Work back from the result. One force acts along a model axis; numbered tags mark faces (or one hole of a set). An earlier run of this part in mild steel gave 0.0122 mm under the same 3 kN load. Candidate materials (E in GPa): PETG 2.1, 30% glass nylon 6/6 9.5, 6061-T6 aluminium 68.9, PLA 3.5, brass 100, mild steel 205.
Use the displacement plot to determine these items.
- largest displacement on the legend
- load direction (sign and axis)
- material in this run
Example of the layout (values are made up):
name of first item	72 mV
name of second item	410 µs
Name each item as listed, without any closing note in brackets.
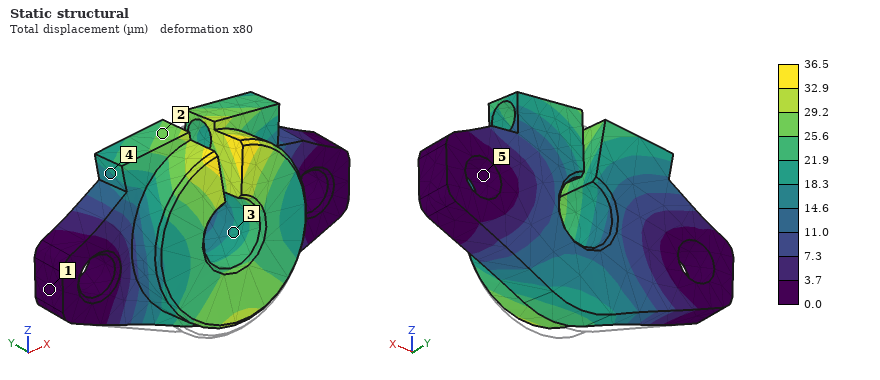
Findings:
largest displacement on the legend	36.5 µm
load direction	+Z
material in this run	6061-T6 aluminium
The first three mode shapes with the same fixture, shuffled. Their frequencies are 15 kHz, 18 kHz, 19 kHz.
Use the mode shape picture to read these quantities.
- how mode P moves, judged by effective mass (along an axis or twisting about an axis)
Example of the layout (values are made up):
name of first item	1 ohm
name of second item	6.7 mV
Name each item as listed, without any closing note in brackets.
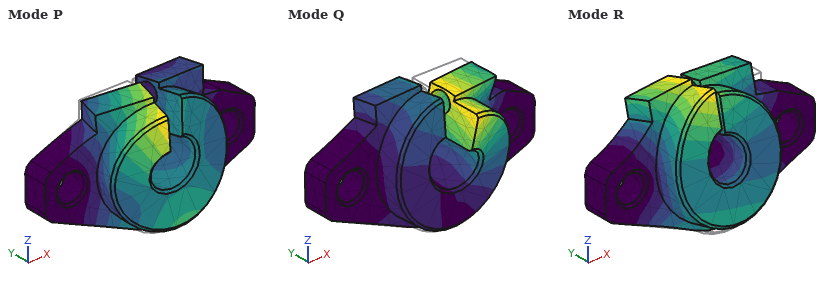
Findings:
how mode P moves, judged by effective mass	along Y
